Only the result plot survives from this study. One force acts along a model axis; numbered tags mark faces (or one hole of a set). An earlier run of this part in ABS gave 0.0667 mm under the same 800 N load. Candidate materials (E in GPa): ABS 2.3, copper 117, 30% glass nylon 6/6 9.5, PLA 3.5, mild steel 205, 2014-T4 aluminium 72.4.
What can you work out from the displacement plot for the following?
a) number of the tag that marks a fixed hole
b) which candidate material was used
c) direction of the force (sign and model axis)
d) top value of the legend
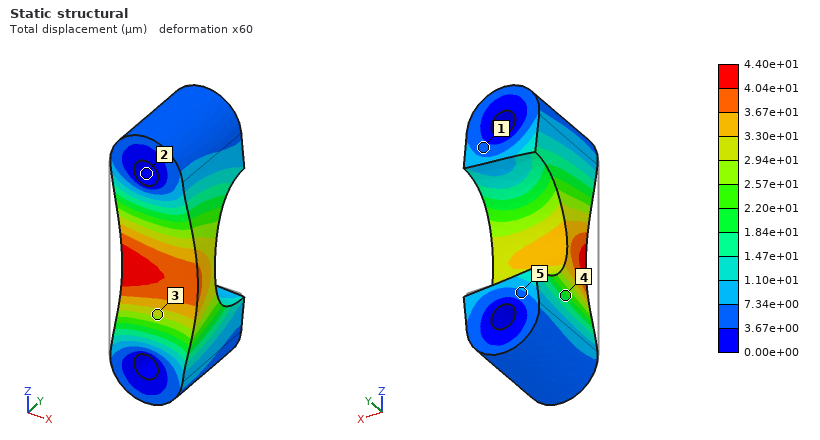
2
PLA
+X
4.40e+01 µm
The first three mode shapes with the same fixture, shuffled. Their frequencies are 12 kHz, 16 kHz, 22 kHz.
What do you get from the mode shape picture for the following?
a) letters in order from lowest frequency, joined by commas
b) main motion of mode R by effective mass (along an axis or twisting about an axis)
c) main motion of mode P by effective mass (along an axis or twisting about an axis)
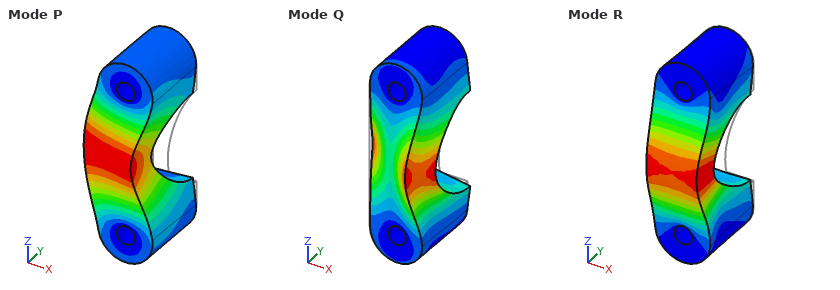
P, R, Q
along Y
along X
